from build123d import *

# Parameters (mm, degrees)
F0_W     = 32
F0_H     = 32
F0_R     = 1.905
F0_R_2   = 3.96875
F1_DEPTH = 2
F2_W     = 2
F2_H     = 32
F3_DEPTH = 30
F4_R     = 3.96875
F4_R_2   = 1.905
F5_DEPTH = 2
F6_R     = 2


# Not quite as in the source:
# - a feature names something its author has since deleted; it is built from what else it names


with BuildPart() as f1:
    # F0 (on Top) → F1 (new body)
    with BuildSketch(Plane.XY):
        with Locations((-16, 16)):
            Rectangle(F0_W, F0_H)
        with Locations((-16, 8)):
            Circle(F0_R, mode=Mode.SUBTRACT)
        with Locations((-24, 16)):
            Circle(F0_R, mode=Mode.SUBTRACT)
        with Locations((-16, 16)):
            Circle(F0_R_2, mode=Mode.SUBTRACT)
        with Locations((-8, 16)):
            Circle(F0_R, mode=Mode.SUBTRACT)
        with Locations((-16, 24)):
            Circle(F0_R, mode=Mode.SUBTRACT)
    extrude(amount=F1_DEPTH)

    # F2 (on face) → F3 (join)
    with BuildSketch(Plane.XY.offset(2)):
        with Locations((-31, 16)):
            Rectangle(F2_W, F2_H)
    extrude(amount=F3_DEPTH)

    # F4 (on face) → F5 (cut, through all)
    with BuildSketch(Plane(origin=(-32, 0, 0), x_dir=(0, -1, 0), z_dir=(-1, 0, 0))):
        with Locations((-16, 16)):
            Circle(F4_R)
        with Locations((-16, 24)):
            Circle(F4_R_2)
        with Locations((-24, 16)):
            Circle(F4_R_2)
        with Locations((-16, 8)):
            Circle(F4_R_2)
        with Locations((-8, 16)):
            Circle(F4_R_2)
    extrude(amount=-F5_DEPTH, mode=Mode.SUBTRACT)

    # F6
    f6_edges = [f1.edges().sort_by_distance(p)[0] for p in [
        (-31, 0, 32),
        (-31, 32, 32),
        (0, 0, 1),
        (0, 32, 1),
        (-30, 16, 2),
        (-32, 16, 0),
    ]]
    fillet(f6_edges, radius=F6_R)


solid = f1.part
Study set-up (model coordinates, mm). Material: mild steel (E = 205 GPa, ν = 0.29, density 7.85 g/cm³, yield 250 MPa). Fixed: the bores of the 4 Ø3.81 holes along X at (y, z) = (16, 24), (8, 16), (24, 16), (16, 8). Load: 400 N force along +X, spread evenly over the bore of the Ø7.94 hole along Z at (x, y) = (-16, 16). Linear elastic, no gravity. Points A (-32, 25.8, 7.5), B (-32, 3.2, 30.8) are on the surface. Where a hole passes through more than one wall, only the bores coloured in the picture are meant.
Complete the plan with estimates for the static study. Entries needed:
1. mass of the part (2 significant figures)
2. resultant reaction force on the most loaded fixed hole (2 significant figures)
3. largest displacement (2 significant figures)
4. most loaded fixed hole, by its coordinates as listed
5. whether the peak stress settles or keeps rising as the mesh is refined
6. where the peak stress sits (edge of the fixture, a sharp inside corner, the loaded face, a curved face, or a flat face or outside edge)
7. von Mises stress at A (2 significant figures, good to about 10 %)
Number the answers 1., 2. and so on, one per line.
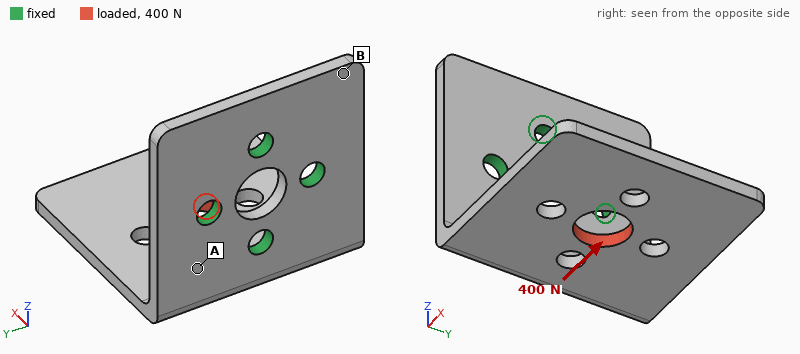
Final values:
1. 28 g
2. 470 N
3. 71 µm
4. (16, 8)
5. keeps rising
6. edge of the fixture
7. 37 MPa
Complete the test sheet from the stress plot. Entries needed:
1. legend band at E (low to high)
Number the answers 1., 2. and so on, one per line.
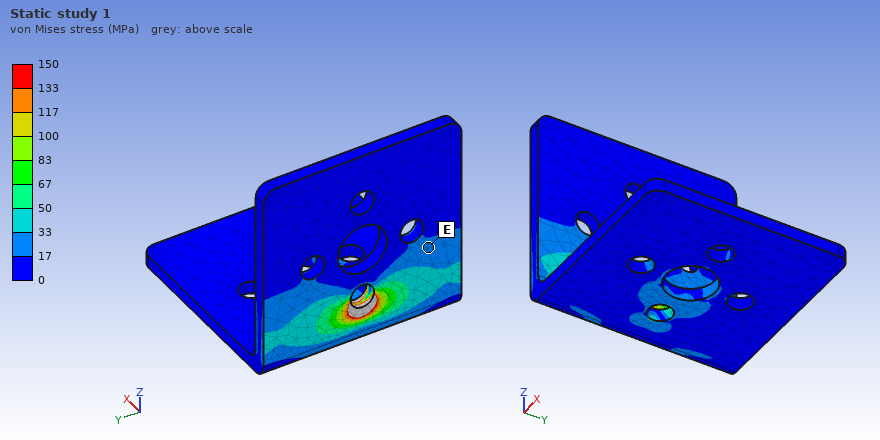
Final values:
1. 17 to 33 MPa
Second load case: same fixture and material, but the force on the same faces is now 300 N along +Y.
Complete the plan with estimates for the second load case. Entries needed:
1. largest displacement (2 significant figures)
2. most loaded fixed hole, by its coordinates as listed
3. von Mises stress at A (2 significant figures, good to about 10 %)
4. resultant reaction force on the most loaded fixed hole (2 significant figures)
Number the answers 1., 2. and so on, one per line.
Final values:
1. 0.10 mm
2. (16, 8)
3. 53 MPa
4. 260 N
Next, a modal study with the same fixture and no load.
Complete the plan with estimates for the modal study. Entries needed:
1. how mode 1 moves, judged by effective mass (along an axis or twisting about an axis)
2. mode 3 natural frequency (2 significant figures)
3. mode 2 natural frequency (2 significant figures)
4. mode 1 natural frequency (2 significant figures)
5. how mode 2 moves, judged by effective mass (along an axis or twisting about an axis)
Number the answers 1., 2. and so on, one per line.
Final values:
1. along Z
2. 3900 Hz
3. 2500 Hz
4. 1400 Hz
5. along Y
